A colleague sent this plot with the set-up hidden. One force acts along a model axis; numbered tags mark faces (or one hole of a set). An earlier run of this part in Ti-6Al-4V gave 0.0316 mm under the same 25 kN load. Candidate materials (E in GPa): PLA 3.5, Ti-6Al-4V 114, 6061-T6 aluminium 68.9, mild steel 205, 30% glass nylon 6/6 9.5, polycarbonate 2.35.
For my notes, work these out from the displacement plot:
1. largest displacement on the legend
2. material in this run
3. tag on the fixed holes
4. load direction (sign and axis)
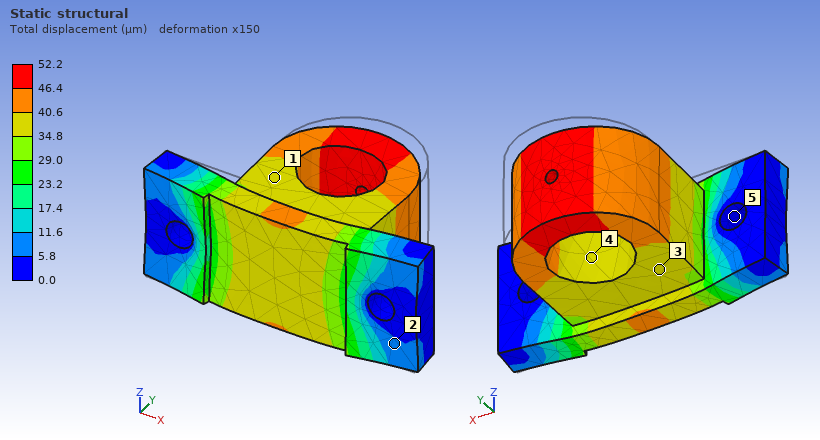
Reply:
52.2 µm
6061-T6 aluminium
5
-Y
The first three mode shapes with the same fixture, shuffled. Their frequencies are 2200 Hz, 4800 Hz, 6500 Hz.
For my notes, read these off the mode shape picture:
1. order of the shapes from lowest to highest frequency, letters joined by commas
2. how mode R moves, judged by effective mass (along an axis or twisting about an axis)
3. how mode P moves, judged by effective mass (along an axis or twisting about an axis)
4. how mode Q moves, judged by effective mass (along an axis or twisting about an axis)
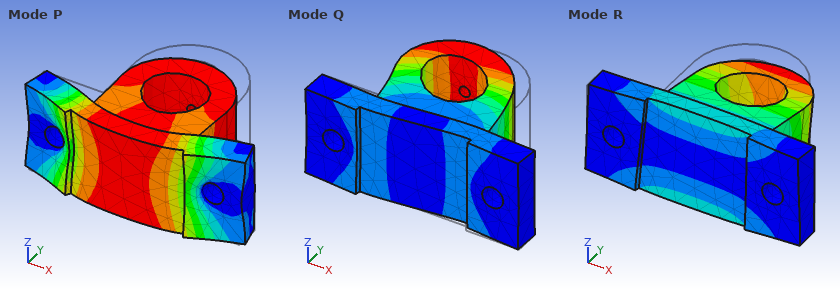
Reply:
R, Q, P
along Z
along Y
along X
